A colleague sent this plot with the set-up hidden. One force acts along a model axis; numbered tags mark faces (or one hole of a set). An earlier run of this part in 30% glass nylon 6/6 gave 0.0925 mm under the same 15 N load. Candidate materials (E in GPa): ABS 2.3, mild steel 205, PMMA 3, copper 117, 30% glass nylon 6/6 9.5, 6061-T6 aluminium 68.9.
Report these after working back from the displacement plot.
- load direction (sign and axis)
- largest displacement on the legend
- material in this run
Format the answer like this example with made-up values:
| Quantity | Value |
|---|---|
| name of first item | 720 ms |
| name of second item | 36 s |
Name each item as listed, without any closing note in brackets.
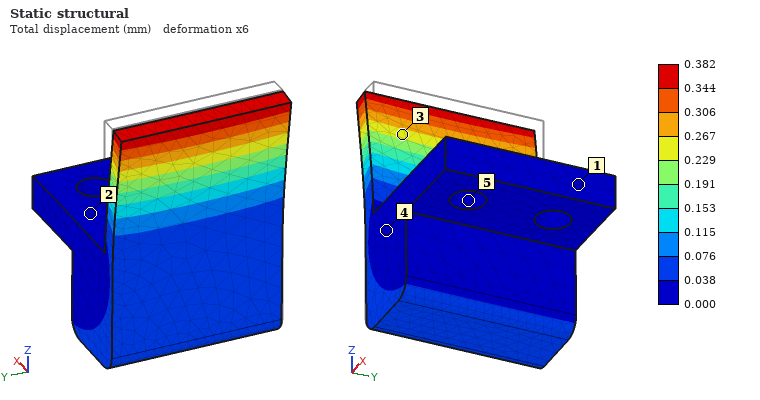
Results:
| Quantity | Value |
|---|---|
| load direction | -X |
| largest displacement on the legend | 0.382 mm |
| material in this run | ABS |
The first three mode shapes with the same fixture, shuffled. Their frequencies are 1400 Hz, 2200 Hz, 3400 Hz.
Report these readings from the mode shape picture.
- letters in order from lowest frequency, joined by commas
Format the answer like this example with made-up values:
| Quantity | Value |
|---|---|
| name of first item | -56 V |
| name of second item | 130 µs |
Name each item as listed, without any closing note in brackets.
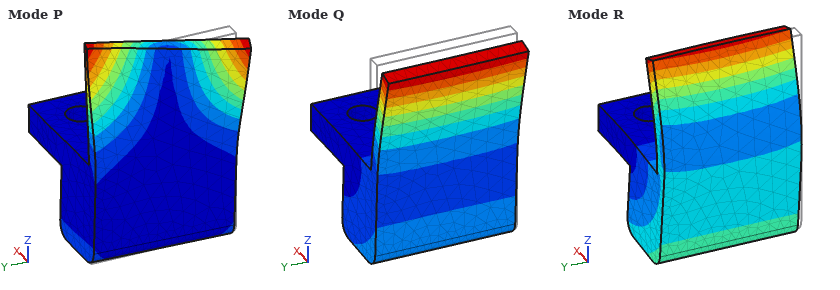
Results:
| Quantity | Value |
|---|---|
| letters in order from lowest frequency, joined by commas | Q, R, P |
